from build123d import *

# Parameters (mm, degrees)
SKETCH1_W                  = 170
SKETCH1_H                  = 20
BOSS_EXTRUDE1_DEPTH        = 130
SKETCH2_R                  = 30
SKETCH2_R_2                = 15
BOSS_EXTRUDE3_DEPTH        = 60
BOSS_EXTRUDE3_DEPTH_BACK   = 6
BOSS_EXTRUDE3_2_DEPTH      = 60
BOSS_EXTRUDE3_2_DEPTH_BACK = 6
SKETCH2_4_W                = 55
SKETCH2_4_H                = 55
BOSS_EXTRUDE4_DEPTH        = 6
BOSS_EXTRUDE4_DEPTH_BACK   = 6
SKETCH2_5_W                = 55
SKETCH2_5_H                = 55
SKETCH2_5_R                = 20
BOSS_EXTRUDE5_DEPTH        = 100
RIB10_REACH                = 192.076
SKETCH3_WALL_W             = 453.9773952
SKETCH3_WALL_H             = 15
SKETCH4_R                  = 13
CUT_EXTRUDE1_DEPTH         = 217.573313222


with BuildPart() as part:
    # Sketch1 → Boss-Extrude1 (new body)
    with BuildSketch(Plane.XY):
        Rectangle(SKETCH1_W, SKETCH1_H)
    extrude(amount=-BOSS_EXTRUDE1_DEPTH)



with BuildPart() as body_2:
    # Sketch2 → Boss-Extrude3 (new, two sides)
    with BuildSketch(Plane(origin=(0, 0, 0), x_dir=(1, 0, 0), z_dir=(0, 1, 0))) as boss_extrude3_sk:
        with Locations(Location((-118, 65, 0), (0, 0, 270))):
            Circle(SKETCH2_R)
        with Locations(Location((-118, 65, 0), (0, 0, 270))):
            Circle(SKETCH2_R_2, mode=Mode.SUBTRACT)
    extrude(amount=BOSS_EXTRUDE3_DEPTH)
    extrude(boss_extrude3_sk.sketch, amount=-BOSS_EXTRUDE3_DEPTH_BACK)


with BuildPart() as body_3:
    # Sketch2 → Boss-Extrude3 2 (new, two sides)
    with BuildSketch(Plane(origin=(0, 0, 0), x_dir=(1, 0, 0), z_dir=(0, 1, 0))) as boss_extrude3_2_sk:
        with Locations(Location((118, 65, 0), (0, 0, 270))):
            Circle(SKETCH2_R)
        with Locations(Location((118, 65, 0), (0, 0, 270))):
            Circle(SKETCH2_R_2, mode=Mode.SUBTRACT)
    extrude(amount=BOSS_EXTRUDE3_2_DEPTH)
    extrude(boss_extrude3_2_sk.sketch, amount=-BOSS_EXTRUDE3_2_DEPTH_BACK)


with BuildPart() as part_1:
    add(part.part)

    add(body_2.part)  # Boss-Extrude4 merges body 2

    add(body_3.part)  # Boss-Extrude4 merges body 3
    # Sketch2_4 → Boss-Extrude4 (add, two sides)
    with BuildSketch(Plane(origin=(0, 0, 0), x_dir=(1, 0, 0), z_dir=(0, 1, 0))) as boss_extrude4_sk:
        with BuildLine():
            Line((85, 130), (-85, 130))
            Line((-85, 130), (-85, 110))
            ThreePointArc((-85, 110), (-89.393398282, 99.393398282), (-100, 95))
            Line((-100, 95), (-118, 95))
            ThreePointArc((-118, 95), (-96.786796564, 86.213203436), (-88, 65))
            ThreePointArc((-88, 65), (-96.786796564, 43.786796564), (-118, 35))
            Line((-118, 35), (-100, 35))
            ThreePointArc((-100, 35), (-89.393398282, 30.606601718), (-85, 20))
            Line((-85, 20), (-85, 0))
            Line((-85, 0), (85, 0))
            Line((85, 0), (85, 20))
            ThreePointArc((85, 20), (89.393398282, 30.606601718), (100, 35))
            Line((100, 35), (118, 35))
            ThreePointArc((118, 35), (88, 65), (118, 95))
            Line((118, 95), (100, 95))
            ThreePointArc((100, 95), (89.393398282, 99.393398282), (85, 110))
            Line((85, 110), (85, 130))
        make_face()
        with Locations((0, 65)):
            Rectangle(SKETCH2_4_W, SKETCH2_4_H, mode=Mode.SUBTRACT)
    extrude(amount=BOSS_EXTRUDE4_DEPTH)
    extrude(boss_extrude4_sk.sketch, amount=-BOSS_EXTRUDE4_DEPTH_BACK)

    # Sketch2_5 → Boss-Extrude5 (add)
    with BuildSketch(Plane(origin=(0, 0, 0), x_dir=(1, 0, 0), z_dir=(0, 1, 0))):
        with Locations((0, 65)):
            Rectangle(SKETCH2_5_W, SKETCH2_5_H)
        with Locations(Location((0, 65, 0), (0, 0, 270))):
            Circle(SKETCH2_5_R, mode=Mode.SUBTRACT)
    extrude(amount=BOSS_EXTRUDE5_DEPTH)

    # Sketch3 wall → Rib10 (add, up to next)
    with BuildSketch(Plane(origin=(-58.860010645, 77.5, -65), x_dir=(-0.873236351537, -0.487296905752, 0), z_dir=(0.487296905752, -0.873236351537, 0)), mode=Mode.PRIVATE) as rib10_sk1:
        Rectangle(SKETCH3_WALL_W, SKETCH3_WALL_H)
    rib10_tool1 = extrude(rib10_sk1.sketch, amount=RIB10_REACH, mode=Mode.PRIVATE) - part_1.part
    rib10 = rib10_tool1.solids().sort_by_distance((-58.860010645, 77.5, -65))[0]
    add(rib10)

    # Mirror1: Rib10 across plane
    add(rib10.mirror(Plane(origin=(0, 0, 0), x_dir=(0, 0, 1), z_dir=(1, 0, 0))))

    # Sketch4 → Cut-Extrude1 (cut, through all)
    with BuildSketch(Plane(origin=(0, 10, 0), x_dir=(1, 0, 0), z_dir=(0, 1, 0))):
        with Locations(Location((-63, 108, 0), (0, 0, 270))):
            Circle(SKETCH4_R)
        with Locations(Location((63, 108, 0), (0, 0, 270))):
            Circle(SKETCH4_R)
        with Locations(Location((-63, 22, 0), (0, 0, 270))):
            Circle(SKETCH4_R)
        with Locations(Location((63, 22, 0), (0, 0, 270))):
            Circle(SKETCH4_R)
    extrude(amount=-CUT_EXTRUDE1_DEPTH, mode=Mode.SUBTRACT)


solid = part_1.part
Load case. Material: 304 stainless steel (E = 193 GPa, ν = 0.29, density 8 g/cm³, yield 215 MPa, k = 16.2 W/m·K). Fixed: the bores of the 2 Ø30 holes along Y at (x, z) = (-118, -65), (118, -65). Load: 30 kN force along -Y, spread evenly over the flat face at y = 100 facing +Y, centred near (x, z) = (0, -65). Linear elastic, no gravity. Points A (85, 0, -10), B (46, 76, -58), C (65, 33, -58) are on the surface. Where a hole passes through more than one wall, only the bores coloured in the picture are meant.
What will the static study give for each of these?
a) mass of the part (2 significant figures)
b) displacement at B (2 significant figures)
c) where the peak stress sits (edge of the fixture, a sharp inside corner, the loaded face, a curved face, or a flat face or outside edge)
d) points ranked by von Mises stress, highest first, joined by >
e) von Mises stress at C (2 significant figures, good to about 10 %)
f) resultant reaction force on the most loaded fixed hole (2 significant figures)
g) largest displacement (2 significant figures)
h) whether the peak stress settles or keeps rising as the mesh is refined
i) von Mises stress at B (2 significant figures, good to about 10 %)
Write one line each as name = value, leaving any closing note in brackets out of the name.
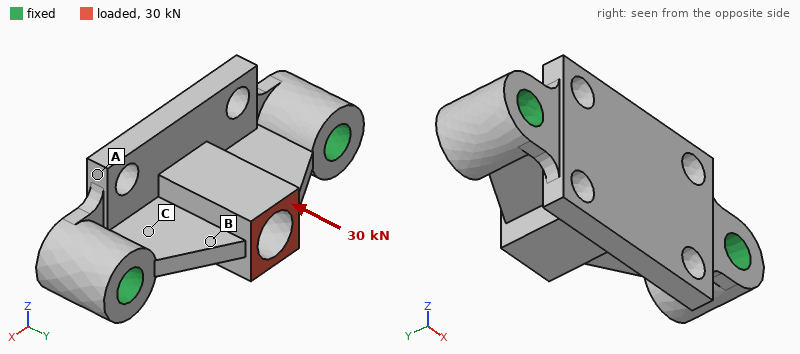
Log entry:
mass of the part = 7.8 kg
displacement at B = 17 µm
where the peak stress sits = a sharp inside corner
points ranked by von Mises stress, highest first, joined by > = C > B > A
von Mises stress at C = 28 MPa
resultant reaction force on the most loaded fixed hole = 15 kN
largest displacement = 29 µm
whether the peak stress settles or keeps rising as the mesh is refined = keeps rising
von Mises stress at B = 13 MPa
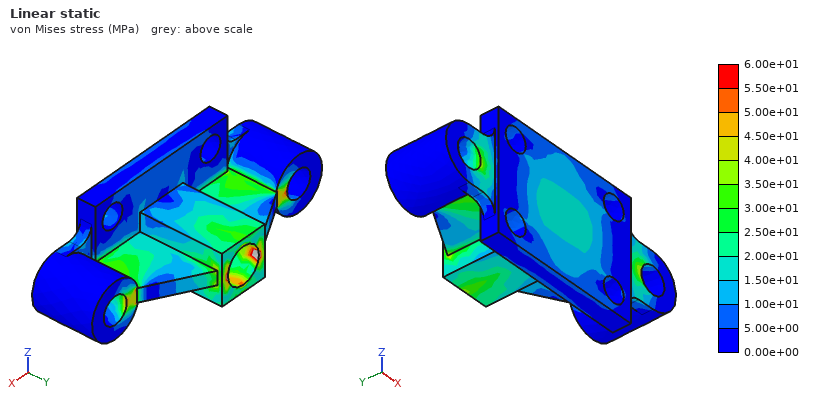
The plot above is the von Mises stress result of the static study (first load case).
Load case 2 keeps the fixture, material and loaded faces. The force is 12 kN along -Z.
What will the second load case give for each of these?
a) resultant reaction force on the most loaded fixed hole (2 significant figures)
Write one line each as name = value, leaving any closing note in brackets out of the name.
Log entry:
resultant reaction force on the most loaded fixed hole = 6.0 kN
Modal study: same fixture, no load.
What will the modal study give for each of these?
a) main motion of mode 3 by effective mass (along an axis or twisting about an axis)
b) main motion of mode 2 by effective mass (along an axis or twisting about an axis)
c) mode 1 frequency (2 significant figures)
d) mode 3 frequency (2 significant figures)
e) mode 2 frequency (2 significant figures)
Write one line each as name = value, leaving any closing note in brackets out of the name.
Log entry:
main motion of mode 3 by effective mass = along Z
main motion of mode 2 by effective mass = along Y
mode 1 frequency = 1500 Hz
mode 3 frequency = 3300 Hz
mode 2 frequency = 2900 Hz
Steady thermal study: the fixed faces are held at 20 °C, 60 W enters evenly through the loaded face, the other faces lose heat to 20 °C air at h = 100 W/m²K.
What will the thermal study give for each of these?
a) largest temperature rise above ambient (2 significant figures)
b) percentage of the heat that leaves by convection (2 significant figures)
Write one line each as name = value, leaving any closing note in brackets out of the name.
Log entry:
largest temperature rise above ambient = 57 K
percentage of the heat that leaves by convection = 97 %
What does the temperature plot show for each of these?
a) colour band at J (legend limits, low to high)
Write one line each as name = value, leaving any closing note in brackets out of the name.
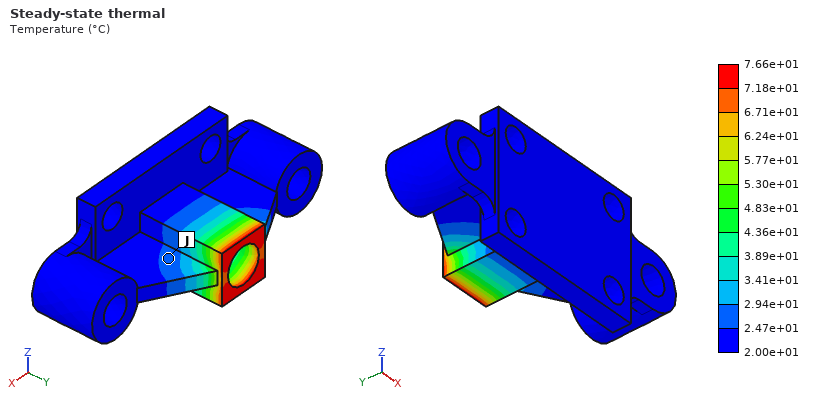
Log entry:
colour band at J = 2.47e+01 to 2.94e+01 °C
